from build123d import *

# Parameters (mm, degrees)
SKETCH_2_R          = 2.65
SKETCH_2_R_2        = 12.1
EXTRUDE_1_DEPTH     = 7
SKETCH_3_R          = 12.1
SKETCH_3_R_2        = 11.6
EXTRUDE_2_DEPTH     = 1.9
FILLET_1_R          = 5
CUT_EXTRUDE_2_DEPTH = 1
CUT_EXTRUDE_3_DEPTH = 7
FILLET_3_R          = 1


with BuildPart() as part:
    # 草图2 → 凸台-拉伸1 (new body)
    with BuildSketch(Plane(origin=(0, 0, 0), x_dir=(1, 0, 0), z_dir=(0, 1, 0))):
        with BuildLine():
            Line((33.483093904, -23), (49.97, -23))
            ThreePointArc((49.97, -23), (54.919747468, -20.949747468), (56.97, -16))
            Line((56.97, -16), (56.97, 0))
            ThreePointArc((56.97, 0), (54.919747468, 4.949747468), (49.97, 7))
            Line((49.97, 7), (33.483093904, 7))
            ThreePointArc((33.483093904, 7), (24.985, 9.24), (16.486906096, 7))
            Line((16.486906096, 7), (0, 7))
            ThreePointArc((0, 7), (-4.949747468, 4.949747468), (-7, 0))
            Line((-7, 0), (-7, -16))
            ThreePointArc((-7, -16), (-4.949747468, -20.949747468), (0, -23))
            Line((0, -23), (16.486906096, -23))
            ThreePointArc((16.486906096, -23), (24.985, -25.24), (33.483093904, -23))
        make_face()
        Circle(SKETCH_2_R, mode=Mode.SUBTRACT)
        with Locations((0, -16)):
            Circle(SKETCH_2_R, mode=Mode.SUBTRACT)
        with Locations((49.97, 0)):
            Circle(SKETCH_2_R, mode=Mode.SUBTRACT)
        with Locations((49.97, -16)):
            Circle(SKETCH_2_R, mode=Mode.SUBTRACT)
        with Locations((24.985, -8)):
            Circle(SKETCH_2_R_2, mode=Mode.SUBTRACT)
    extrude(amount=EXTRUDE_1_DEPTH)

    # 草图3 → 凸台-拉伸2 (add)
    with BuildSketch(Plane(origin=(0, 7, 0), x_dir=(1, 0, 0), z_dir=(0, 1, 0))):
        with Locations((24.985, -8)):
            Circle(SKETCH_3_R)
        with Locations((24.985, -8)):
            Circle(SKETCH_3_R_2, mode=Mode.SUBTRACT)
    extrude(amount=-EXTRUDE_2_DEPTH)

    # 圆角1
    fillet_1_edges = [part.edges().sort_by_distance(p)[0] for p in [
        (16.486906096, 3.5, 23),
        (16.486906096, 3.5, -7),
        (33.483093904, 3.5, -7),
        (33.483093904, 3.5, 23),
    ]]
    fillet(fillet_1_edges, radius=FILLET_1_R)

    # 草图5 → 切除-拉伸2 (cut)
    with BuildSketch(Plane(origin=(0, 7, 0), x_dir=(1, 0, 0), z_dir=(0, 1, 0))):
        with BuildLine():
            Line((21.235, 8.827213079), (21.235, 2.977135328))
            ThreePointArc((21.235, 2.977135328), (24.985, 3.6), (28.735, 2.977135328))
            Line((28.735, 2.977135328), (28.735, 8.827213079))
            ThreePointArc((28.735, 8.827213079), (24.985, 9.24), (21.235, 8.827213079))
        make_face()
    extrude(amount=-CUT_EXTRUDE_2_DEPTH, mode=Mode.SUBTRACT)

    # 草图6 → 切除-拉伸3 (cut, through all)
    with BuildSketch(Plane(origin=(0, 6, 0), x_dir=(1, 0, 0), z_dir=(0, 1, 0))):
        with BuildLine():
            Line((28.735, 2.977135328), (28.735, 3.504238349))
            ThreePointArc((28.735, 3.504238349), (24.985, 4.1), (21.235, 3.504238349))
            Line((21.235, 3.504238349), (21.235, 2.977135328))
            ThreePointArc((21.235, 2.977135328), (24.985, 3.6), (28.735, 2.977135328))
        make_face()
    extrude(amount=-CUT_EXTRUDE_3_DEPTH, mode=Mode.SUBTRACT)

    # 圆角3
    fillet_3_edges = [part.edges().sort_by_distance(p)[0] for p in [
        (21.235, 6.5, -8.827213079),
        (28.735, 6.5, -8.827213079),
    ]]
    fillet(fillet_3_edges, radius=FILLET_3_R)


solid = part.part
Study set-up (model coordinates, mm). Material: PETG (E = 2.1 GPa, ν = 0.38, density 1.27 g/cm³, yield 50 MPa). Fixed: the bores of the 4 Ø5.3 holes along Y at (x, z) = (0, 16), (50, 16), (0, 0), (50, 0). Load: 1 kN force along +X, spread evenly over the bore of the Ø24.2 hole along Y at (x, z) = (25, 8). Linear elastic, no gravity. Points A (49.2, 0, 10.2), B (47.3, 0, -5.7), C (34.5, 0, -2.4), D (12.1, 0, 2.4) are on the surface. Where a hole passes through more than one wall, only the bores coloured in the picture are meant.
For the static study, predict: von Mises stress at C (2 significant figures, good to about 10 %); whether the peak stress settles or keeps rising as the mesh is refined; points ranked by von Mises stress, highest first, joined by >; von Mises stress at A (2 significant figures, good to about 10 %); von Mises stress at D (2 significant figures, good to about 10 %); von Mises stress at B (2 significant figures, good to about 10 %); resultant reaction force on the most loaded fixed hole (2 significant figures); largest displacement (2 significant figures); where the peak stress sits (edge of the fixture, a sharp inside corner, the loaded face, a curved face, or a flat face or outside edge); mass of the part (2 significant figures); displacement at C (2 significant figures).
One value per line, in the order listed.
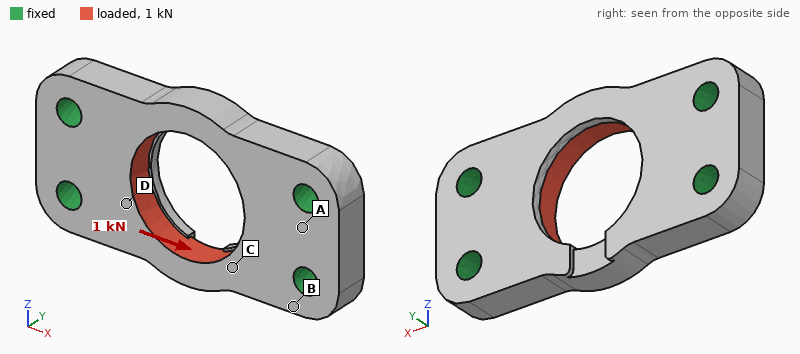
4.3 MPa
keeps rising
C > D > B > A
1.0 MPa
3.3 MPa
1.8 MPa
260 N
39 µm
a sharp inside corner
12 g
28 µm
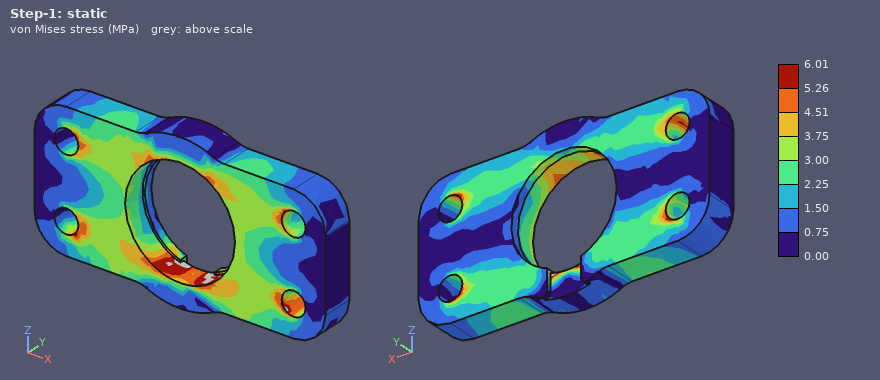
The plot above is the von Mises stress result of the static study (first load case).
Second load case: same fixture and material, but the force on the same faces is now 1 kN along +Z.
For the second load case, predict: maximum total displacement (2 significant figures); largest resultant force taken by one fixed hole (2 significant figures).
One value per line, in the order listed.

0.15 mm
300 N
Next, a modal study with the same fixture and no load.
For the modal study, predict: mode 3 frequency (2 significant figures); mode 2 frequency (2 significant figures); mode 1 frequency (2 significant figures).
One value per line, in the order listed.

8100 Hz
4300 Hz
4200 Hz
